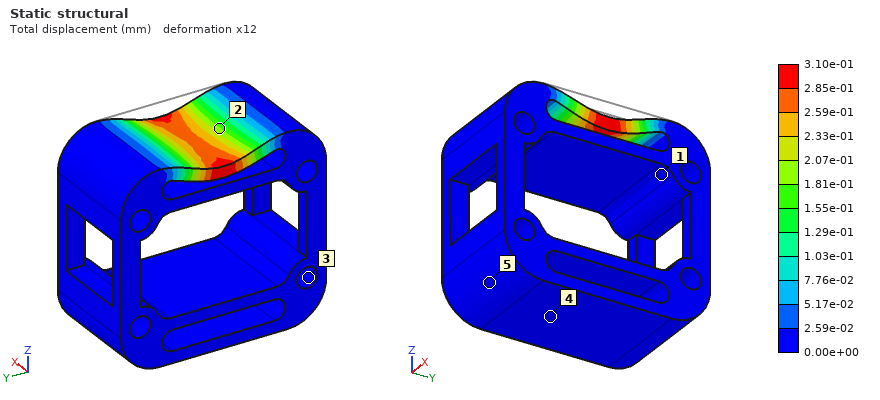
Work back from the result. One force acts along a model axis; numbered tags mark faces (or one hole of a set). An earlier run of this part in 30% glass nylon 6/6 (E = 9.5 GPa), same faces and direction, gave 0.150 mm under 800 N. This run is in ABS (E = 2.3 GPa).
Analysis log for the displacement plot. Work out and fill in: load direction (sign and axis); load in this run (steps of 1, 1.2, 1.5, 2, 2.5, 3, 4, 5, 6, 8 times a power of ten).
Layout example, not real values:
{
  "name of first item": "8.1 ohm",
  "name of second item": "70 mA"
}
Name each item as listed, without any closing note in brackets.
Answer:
{
  "load direction": "-Z",
  "load in this run": "400 N"
}
